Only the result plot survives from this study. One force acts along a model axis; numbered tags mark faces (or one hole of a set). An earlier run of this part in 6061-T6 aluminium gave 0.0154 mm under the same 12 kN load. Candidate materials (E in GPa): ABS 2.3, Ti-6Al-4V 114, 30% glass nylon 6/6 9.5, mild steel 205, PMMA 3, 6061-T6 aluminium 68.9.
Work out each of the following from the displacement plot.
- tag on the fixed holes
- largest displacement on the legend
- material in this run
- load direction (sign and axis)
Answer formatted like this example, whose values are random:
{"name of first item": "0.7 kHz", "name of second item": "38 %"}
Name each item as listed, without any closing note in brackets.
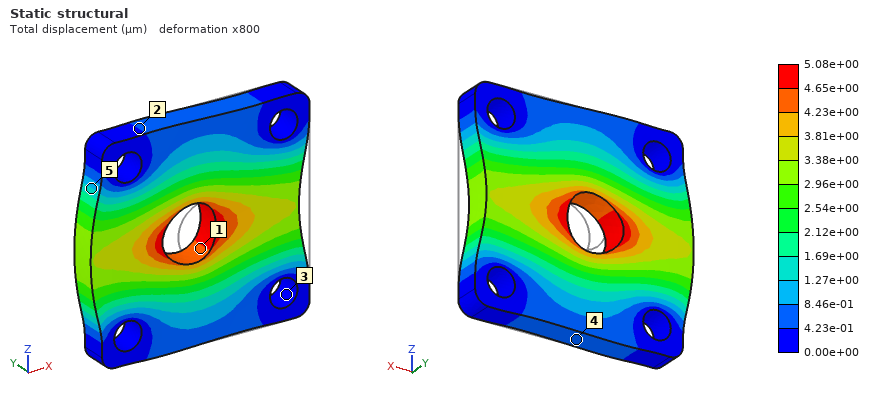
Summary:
{"tag on the fixed holes": "3", "largest displacement on the legend": "5.08e+00 µm", "material in this run": "mild steel", "load direction": "-X"}
